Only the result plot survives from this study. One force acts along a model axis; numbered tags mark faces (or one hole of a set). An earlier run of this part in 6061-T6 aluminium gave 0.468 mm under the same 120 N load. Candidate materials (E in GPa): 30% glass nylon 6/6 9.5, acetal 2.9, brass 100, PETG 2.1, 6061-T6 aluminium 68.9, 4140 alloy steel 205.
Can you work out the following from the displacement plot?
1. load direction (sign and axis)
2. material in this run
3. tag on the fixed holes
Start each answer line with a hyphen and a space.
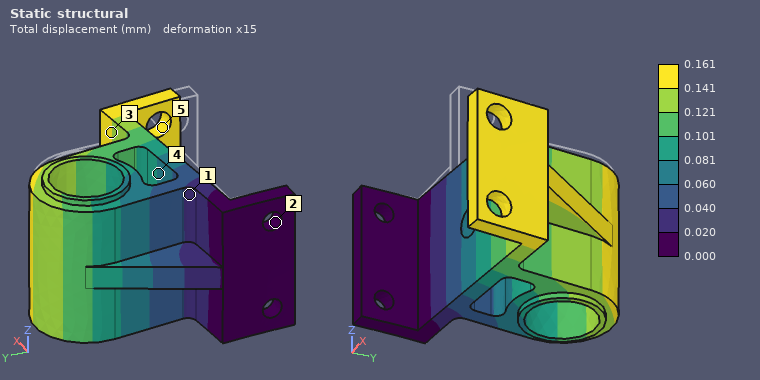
- +Y
- 4140 alloy steel
- 2
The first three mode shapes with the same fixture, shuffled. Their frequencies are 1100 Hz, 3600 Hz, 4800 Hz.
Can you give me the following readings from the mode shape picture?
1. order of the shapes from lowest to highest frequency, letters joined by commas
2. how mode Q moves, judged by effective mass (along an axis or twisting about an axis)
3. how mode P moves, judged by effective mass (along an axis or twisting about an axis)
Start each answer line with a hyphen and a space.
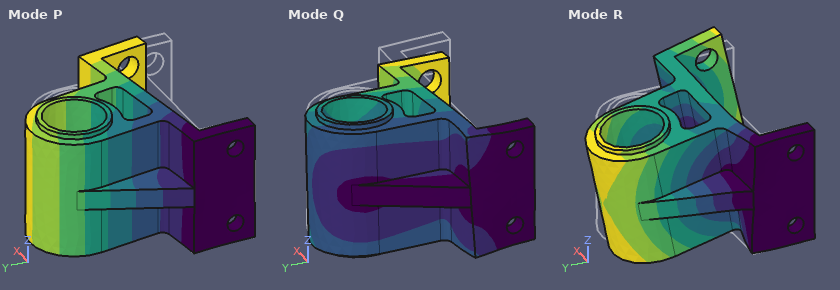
- P, Q, R
- along Z
- along Y
